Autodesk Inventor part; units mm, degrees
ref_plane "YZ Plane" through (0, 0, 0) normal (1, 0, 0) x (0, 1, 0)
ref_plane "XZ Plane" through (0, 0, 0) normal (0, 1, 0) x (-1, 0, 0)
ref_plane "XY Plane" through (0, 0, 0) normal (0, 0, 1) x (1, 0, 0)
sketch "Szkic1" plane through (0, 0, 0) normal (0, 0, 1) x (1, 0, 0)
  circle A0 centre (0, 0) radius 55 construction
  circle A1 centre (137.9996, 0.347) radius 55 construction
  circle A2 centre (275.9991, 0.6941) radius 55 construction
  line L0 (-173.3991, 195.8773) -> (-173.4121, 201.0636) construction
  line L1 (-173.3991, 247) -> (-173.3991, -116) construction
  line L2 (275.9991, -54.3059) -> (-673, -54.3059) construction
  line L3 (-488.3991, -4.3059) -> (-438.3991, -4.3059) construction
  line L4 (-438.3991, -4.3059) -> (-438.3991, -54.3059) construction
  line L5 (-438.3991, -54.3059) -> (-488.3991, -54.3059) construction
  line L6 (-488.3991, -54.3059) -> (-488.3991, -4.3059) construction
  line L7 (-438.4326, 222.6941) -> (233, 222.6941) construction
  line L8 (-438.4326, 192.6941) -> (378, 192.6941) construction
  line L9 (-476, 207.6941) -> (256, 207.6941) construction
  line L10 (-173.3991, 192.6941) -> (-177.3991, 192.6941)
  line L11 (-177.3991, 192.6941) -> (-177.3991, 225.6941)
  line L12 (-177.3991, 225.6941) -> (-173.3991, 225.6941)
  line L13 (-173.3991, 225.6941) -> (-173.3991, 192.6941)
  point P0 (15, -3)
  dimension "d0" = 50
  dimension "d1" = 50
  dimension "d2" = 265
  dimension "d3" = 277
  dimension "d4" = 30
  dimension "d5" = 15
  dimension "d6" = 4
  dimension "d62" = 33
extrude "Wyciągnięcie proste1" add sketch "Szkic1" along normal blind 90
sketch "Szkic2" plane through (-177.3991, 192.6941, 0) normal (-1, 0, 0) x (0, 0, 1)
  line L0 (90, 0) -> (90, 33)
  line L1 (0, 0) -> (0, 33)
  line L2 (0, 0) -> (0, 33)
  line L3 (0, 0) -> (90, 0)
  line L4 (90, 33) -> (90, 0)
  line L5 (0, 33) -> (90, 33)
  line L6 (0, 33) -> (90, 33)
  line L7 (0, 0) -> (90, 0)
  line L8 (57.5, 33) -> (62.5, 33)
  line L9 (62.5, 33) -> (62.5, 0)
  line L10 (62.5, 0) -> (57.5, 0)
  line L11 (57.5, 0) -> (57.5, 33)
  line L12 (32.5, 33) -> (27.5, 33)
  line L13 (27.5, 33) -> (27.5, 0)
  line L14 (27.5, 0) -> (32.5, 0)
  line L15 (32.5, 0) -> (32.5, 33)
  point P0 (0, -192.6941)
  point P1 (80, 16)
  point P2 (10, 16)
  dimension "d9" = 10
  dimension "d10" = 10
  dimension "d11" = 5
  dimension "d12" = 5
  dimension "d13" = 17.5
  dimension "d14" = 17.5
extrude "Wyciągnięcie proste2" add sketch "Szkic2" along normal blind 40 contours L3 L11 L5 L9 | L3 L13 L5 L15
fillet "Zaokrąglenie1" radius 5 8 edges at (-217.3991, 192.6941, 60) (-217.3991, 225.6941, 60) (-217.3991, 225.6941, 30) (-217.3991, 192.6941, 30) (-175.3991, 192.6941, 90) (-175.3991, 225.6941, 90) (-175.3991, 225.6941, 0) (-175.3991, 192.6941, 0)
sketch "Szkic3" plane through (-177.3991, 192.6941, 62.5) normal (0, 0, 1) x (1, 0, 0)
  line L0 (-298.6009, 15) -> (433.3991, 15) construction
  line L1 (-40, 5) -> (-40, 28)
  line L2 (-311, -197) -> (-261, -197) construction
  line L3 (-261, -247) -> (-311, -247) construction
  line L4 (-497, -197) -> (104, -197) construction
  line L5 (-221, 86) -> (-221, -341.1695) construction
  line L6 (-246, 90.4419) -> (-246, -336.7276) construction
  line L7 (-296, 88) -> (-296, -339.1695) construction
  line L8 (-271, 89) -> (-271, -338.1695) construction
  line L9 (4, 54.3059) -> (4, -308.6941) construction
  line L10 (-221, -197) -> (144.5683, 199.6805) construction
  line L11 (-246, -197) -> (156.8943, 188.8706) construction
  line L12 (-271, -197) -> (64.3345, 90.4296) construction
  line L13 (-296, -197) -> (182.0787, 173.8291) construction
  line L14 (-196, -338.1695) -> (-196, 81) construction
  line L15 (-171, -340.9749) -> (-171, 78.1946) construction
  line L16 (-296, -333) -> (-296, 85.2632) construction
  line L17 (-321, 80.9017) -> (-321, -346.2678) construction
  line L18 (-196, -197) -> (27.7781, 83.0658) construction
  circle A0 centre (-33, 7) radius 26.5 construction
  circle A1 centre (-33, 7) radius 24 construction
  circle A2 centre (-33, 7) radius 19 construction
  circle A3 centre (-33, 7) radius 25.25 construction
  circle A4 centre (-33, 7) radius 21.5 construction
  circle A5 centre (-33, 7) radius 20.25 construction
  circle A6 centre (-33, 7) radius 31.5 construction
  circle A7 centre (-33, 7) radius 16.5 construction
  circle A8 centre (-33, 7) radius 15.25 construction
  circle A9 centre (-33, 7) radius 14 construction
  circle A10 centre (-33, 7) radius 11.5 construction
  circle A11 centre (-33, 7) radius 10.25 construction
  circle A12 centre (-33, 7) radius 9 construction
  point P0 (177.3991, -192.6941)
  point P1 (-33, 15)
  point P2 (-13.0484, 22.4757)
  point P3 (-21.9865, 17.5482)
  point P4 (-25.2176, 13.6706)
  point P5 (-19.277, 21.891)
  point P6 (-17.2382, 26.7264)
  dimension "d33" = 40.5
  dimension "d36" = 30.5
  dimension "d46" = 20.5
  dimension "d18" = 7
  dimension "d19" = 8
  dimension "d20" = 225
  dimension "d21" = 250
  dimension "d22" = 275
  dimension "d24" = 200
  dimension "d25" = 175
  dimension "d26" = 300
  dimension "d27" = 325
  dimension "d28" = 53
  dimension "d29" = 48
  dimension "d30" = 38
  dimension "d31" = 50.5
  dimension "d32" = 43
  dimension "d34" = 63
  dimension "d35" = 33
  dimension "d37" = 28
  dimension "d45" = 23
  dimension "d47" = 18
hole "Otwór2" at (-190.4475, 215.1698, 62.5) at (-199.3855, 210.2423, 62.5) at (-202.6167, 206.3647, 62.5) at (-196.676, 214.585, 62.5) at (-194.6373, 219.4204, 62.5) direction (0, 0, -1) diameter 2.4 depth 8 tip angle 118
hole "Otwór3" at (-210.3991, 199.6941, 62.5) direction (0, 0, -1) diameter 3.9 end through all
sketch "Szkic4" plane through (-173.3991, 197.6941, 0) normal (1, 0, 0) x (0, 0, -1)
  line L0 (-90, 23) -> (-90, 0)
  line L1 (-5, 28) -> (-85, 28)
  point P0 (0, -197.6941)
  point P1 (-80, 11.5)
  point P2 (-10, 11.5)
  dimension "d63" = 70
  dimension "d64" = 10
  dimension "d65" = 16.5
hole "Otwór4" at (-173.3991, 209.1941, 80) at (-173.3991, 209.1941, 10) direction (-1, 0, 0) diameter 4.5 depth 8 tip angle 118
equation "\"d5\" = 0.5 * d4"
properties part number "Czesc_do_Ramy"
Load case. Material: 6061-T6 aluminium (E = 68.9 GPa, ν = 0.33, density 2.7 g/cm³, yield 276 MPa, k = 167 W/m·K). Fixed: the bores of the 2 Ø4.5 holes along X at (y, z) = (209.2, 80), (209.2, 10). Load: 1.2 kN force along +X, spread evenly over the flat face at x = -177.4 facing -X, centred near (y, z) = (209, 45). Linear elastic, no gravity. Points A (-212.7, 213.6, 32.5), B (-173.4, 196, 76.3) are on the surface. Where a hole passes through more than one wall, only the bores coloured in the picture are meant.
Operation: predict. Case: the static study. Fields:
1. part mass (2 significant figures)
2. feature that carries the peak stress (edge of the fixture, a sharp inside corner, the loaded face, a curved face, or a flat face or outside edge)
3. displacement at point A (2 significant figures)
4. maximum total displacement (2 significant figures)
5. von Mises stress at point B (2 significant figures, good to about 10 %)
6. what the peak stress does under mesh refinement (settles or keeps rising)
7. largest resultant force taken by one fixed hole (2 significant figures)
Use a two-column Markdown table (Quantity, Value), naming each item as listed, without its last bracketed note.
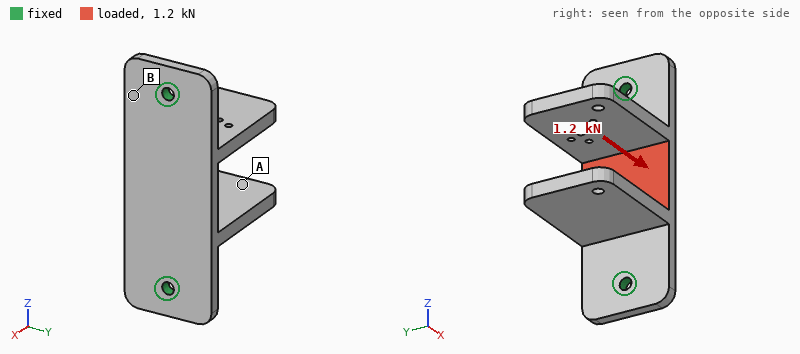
| Quantity | Value |
|---|---|
| part mass | 66 g |
| feature that carries the peak stress | edge of the fixture |
| displacement at point A | 0.28 mm |
| maximum total displacement | 0.31 mm |
| von Mises stress at point B | 44 MPa |
| what the peak stress does under mesh refinement | keeps rising |
| largest resultant force taken by one fixed hole | 600 N |
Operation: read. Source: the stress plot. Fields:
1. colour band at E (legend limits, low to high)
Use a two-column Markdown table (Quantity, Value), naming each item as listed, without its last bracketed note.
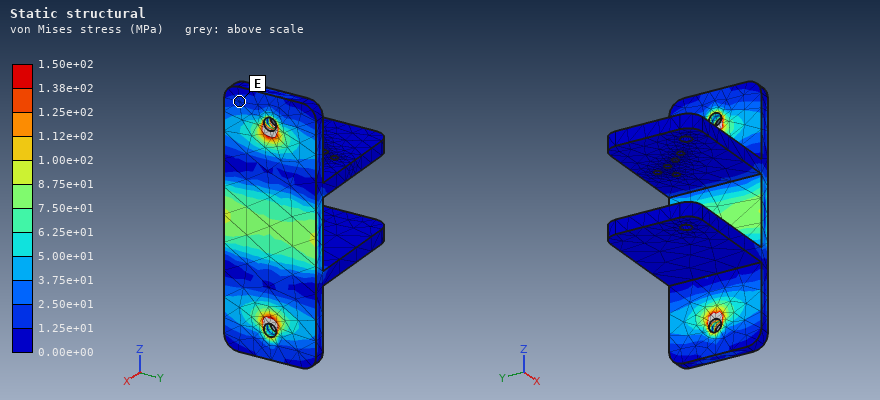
| Quantity | Value |
|---|---|
| colour band at E | 1.25e+01 to 2.50e+01 MPa |
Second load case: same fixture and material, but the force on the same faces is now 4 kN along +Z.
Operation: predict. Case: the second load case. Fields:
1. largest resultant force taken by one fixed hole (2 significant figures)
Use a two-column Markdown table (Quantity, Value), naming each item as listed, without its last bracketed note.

| Quantity | Value |
|---|---|
| largest resultant force taken by one fixed hole | 2.0 kN |
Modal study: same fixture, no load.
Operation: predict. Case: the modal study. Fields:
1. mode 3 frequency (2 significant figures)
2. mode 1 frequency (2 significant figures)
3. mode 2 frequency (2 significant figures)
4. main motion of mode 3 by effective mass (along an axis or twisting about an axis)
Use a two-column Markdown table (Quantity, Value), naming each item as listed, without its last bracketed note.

| Quantity | Value |
|---|---|
| mode 3 frequency | 2100 Hz |
| mode 1 frequency | 1400 Hz |
| mode 2 frequency | 1500 Hz |
| main motion of mode 3 by effective mass | along Z |
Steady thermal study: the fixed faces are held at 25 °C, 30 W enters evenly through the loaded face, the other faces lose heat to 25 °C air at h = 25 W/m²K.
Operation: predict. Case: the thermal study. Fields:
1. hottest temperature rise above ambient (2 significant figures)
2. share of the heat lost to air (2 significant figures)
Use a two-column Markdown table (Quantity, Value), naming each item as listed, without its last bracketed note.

| Quantity | Value |
|---|---|
| hottest temperature rise above ambient | 20 K |
| share of the heat lost to air | 12 % |
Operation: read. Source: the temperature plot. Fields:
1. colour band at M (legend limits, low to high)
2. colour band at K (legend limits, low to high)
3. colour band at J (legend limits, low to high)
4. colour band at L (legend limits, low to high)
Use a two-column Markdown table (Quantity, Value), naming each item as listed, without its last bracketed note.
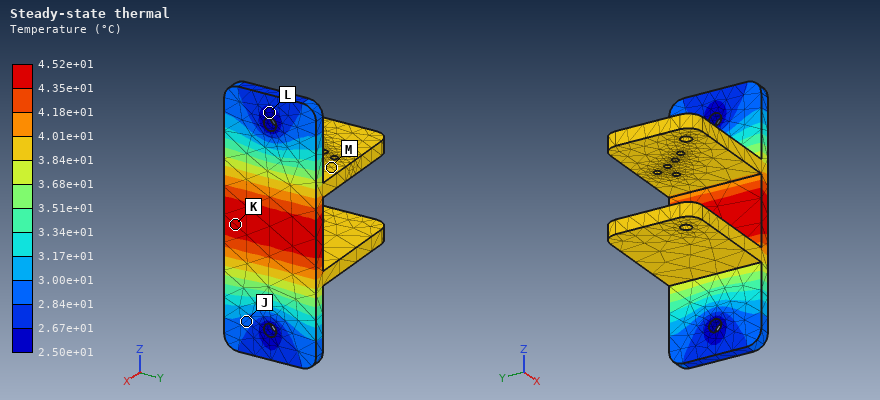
| Quantity | Value |
|---|---|
| colour band at M | 3.84e+01 to 4.01e+01 °C |
| colour band at K | 4.35e+01 to 4.52e+01 °C |
| colour band at J | 2.84e+01 to 3.00e+01 °C |
| colour band at L | 2.50e+01 to 2.67e+01 °C |
